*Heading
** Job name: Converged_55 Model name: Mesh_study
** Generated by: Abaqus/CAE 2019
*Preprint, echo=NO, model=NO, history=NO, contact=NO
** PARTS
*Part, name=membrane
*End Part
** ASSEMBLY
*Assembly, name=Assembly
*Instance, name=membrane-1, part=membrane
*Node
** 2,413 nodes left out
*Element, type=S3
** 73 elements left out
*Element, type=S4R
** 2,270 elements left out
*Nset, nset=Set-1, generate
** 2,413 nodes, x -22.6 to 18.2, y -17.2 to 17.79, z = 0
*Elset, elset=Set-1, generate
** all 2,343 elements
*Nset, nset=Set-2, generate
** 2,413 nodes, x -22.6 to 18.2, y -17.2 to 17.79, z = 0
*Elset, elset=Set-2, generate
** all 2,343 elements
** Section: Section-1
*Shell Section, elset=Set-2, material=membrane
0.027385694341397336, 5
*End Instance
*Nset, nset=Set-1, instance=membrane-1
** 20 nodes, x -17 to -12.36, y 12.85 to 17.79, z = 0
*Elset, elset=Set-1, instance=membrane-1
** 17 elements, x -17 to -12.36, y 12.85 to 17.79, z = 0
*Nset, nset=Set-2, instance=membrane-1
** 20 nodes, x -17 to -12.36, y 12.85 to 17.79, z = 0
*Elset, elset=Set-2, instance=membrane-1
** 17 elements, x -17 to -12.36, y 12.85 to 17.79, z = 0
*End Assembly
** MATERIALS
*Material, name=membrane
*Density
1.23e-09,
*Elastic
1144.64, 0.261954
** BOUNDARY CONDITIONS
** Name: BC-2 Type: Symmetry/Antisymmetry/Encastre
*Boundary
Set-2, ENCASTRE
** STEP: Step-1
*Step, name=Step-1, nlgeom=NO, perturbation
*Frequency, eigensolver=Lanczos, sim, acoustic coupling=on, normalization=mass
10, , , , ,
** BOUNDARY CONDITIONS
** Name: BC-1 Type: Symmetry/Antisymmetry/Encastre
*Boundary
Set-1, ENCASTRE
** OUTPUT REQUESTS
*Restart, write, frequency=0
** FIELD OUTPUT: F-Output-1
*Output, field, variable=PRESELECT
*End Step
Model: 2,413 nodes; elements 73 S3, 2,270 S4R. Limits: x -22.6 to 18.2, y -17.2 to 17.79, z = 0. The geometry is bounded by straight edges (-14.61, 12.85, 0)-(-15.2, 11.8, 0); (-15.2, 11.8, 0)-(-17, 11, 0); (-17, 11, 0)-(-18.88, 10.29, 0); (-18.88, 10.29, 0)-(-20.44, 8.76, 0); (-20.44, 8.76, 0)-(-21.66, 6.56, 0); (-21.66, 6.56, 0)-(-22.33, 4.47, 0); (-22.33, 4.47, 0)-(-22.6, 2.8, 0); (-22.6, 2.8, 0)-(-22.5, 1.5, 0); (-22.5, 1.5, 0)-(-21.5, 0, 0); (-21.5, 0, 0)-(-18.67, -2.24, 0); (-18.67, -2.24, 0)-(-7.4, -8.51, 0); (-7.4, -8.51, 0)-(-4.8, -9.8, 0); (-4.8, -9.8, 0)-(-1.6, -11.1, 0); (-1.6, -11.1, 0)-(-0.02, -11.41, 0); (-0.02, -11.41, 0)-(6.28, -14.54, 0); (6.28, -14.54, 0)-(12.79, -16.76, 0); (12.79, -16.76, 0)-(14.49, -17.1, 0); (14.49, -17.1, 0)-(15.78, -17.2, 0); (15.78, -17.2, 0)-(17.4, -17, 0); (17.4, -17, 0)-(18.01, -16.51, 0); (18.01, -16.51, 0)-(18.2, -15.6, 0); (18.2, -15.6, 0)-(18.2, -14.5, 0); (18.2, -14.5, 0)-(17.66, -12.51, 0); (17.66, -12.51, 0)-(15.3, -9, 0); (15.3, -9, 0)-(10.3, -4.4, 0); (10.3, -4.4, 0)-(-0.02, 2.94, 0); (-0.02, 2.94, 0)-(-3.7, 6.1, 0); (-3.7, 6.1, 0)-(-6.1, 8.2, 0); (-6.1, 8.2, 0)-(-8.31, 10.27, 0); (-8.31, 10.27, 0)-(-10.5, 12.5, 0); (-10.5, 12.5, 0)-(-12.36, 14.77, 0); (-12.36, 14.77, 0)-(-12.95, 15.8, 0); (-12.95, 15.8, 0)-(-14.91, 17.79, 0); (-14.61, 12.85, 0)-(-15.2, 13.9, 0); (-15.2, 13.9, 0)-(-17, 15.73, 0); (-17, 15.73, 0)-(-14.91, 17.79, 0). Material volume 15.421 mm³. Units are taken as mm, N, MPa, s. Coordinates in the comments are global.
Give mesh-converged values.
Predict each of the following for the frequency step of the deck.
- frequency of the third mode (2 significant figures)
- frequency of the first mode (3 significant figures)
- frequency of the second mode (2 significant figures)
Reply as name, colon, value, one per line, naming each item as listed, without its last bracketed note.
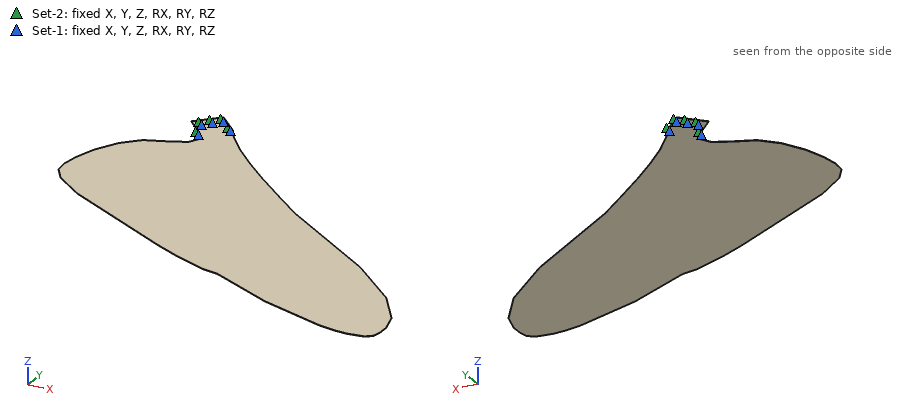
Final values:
frequency of the third mode: 18 Hz
frequency of the first mode: 2.15 Hz
frequency of the second mode: 9.2 Hz
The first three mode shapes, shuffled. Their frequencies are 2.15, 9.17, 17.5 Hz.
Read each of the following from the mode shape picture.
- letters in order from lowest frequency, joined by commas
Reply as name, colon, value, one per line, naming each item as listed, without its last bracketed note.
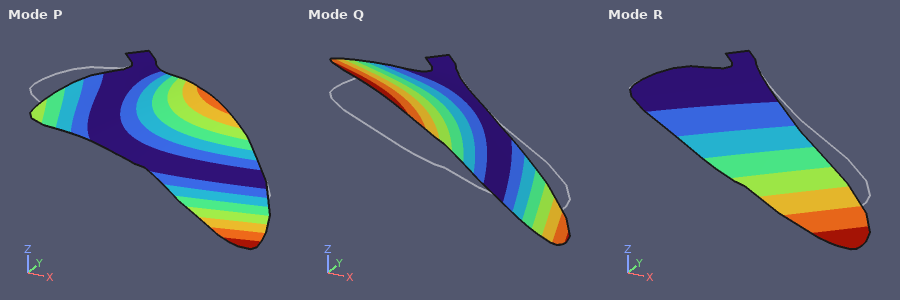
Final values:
letters in order from lowest frequency, joined by commas: R, Q, P
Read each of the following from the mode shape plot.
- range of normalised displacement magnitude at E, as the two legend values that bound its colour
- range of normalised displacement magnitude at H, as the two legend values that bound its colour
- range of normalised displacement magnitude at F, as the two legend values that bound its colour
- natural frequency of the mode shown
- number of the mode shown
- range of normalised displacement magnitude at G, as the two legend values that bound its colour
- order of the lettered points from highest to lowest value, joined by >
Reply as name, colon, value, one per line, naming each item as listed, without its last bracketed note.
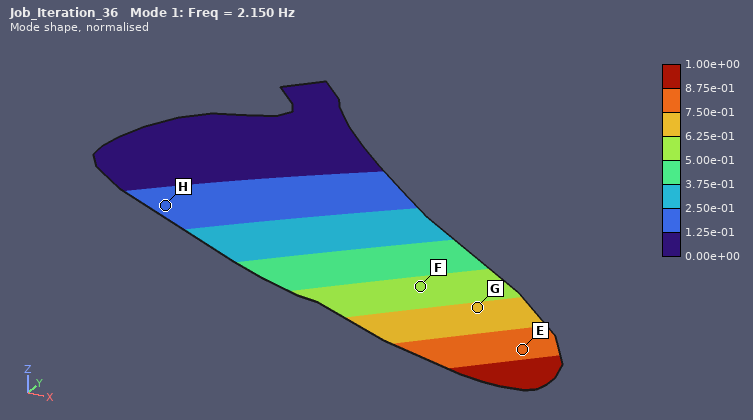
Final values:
range of normalised displacement magnitude at E, as the two legend values that bound its colour: 7.50e-01 to 8.75e-01
range of normalised displacement magnitude at H, as the two legend values that bound its colour: 1.25e-01 to 2.50e-01
range of normalised displacement magnitude at F, as the two legend values that bound its colour: 5.00e-01 to 6.25e-01
natural frequency of the mode shown: 2.150 Hz
number of the mode shown: 1
range of normalised displacement magnitude at G, as the two legend values that bound its colour: 6.25e-01 to 7.50e-01
order of the lettered points from highest to lowest value, joined by >: E > G > F > H
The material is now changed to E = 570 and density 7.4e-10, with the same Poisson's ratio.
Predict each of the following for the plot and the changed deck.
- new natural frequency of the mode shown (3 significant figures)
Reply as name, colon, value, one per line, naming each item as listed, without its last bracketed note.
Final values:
new natural frequency of the mode shown: 1.96 Hz
